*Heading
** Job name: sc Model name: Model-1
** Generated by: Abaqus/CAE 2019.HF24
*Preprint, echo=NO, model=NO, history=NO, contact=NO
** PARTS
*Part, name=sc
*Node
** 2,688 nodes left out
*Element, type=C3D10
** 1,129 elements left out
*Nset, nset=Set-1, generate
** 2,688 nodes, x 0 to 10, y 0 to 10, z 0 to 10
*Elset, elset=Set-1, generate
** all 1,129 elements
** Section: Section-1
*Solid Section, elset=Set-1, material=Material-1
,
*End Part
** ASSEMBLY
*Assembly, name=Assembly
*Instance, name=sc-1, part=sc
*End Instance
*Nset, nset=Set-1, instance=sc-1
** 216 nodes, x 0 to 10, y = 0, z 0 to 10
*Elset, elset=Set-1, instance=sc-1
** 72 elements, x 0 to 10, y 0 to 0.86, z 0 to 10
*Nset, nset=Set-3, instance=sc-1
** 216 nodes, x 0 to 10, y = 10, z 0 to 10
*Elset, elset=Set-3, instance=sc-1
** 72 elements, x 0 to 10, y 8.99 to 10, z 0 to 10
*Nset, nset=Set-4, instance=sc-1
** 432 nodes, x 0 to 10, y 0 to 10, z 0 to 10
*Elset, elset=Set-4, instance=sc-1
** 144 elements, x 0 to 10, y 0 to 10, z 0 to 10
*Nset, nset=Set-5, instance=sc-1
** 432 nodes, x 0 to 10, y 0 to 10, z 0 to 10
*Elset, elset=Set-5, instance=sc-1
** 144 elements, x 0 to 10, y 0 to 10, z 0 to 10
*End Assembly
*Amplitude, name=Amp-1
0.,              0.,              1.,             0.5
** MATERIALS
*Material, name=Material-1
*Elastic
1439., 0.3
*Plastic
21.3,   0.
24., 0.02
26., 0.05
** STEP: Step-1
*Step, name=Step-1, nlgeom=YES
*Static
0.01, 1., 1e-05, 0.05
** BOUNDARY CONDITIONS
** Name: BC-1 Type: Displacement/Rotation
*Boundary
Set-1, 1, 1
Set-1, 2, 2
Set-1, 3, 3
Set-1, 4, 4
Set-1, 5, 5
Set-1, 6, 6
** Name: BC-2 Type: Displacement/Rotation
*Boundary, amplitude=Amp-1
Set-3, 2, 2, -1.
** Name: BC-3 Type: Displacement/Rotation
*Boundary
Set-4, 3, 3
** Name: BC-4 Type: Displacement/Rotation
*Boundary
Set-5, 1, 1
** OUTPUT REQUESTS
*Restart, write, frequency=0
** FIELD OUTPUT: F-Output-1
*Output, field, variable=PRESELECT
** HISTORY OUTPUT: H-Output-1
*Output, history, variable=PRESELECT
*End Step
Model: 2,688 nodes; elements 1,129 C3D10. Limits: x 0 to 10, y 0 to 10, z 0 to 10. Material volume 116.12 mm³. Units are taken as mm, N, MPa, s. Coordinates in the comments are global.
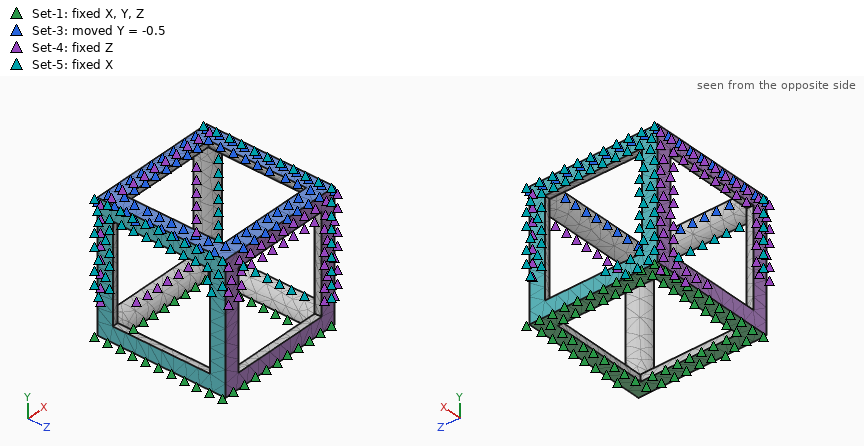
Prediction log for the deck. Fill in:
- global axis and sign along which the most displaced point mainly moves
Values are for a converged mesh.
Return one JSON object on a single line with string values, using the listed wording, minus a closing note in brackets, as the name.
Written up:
{"global axis and sign along which the most displaced point mainly moves": "-Y"}
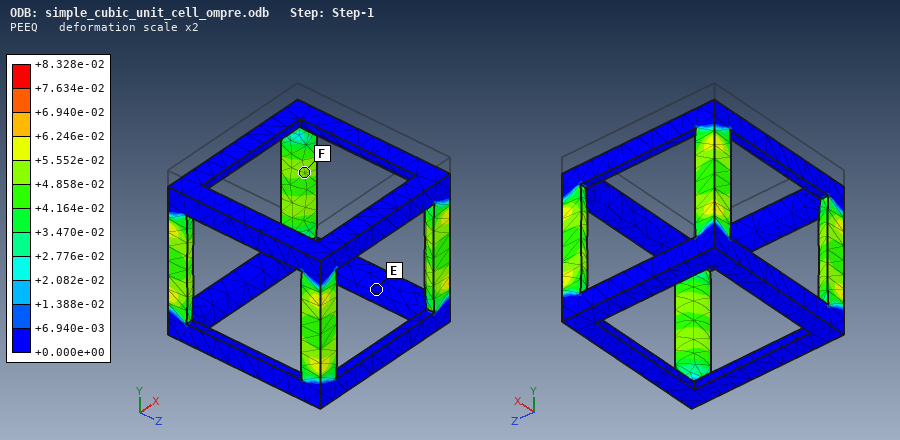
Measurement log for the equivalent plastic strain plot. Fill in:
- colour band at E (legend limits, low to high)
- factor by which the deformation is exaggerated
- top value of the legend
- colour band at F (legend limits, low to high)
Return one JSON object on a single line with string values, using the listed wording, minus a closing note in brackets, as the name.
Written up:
{"colour band at E": "+0.000e+00 to +6.940e-03", "factor by which the deformation is exaggerated": "2", "top value of the legend": "+8.328e-02", "colour band at F": "+4.858e-02 to +5.552e-02"}
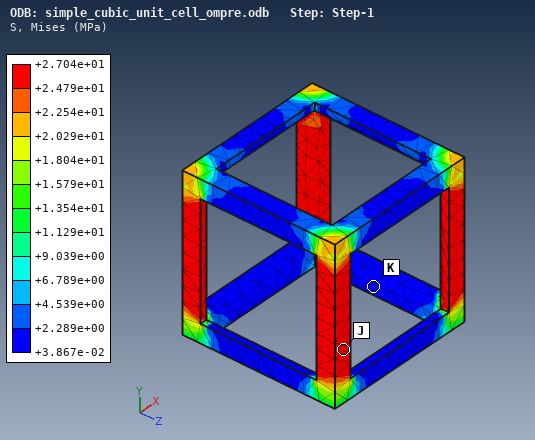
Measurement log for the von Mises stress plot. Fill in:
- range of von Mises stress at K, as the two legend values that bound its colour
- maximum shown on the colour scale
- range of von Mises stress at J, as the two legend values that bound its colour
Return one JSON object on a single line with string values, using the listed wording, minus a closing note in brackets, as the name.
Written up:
{"range of von Mises stress at K, as the two legend values that bound its colour": "+3.867e-02 to +2.289e+00 MPa", "maximum shown on the colour scale": "+2.704e+01 MPa", "range of von Mises stress at J, as the two legend values that bound its colour": "+2.479e+01 to +2.704e+01 MPa"}
